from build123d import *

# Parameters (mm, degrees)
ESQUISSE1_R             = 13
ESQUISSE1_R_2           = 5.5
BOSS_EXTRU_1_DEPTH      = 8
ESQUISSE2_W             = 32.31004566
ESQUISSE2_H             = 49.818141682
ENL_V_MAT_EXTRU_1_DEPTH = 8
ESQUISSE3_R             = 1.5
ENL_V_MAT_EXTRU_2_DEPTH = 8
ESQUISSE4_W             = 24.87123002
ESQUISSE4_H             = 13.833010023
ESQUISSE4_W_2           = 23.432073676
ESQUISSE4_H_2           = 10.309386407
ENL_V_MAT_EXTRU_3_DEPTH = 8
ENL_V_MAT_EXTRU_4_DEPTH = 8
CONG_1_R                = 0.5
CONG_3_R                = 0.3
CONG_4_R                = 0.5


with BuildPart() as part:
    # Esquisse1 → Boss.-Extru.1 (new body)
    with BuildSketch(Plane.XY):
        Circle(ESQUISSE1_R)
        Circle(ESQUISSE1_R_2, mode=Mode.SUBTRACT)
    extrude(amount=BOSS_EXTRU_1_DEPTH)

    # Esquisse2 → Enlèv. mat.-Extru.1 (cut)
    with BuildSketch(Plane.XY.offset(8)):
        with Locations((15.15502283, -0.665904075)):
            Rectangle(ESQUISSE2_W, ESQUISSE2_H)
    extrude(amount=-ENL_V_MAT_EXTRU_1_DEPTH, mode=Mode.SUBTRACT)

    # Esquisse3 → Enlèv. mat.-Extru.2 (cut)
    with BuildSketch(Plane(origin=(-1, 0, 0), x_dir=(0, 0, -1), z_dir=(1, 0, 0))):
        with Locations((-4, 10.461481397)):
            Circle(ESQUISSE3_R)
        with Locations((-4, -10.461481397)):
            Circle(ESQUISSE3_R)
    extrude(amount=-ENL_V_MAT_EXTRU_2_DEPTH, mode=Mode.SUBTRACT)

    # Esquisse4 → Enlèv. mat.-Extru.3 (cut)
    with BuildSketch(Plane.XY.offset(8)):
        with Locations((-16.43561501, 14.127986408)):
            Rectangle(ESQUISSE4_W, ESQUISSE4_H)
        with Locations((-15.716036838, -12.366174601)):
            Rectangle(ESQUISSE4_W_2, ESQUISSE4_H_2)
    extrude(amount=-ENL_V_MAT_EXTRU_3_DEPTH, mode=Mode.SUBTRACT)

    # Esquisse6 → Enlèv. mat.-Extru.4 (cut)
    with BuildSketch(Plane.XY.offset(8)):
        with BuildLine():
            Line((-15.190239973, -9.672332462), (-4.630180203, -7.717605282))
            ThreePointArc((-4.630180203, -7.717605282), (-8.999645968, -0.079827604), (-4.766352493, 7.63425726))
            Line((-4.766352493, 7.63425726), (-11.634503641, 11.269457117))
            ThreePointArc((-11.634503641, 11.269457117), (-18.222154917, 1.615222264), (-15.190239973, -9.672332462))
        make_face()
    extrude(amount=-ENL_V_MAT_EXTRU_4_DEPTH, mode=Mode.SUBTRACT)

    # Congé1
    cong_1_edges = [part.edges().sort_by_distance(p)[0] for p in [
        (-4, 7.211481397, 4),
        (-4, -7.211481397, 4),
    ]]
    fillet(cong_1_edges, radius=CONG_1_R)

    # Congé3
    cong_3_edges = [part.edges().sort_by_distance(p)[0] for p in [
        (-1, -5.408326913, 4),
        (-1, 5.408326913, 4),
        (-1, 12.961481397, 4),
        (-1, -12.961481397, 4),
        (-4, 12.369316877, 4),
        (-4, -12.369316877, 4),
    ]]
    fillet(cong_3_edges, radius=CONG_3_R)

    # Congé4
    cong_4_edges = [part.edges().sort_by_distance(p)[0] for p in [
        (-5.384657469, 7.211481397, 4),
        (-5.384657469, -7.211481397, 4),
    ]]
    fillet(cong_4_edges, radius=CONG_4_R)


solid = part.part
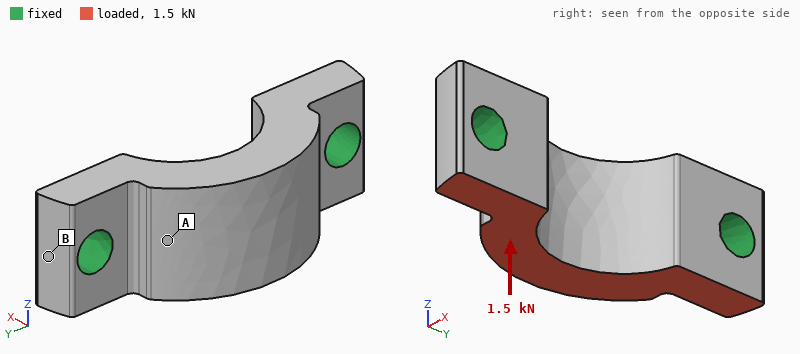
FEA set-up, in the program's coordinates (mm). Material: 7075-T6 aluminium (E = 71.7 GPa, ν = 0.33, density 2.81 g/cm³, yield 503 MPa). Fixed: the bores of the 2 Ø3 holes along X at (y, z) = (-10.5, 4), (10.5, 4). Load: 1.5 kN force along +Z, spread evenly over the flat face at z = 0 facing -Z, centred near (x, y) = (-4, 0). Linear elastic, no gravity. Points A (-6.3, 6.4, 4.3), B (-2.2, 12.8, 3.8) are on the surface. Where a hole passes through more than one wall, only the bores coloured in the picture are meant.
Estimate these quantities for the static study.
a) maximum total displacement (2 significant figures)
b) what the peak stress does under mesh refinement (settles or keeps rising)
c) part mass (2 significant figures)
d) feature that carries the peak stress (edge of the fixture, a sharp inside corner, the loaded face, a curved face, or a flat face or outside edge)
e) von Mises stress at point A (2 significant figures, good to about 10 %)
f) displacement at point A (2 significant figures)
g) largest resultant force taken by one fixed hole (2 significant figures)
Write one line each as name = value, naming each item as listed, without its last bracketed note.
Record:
maximum total displacement = 35 µm
what the peak stress does under mesh refinement = keeps rising
part mass = 2.0 g
feature that carries the peak stress = edge of the fixture
von Mises stress at point A = 58 MPa
displacement at point A = 18 µm
largest resultant force taken by one fixed hole = 750 N
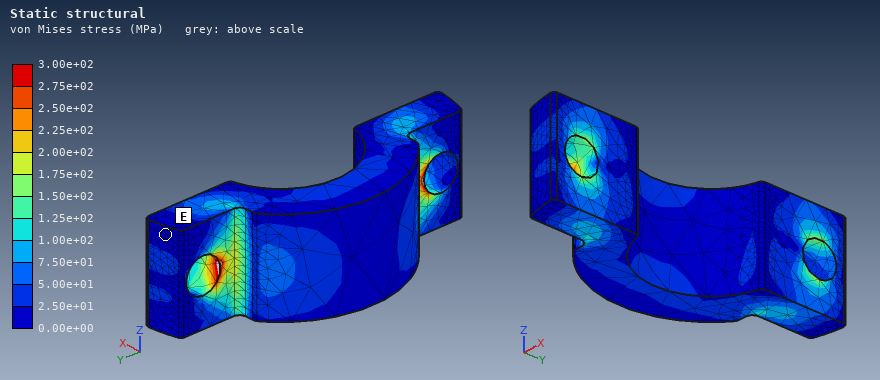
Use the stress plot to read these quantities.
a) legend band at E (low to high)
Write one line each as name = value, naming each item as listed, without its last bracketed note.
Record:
legend band at E = 0.00e+00 to 2.50e+01 MPa
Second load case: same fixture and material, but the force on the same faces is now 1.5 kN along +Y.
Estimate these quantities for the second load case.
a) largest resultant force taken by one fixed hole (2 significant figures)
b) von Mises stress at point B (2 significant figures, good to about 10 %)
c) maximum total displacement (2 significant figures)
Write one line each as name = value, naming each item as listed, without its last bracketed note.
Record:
largest resultant force taken by one fixed hole = 790 N
von Mises stress at point B = 32 MPa
maximum total displacement = 10 µm
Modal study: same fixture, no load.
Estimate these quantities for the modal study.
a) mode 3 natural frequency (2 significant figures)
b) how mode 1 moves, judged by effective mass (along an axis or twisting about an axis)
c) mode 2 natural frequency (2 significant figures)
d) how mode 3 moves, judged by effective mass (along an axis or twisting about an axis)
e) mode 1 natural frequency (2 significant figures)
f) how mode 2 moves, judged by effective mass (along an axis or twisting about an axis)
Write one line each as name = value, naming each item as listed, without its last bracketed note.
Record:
mode 3 natural frequency = 66 kHz
how mode 1 moves, judged by effective mass = along Z
mode 2 natural frequency = 50 kHz
how mode 3 moves, judged by effective mass = along Y
mode 1 natural frequency = 27 kHz
how mode 2 moves, judged by effective mass = along X
